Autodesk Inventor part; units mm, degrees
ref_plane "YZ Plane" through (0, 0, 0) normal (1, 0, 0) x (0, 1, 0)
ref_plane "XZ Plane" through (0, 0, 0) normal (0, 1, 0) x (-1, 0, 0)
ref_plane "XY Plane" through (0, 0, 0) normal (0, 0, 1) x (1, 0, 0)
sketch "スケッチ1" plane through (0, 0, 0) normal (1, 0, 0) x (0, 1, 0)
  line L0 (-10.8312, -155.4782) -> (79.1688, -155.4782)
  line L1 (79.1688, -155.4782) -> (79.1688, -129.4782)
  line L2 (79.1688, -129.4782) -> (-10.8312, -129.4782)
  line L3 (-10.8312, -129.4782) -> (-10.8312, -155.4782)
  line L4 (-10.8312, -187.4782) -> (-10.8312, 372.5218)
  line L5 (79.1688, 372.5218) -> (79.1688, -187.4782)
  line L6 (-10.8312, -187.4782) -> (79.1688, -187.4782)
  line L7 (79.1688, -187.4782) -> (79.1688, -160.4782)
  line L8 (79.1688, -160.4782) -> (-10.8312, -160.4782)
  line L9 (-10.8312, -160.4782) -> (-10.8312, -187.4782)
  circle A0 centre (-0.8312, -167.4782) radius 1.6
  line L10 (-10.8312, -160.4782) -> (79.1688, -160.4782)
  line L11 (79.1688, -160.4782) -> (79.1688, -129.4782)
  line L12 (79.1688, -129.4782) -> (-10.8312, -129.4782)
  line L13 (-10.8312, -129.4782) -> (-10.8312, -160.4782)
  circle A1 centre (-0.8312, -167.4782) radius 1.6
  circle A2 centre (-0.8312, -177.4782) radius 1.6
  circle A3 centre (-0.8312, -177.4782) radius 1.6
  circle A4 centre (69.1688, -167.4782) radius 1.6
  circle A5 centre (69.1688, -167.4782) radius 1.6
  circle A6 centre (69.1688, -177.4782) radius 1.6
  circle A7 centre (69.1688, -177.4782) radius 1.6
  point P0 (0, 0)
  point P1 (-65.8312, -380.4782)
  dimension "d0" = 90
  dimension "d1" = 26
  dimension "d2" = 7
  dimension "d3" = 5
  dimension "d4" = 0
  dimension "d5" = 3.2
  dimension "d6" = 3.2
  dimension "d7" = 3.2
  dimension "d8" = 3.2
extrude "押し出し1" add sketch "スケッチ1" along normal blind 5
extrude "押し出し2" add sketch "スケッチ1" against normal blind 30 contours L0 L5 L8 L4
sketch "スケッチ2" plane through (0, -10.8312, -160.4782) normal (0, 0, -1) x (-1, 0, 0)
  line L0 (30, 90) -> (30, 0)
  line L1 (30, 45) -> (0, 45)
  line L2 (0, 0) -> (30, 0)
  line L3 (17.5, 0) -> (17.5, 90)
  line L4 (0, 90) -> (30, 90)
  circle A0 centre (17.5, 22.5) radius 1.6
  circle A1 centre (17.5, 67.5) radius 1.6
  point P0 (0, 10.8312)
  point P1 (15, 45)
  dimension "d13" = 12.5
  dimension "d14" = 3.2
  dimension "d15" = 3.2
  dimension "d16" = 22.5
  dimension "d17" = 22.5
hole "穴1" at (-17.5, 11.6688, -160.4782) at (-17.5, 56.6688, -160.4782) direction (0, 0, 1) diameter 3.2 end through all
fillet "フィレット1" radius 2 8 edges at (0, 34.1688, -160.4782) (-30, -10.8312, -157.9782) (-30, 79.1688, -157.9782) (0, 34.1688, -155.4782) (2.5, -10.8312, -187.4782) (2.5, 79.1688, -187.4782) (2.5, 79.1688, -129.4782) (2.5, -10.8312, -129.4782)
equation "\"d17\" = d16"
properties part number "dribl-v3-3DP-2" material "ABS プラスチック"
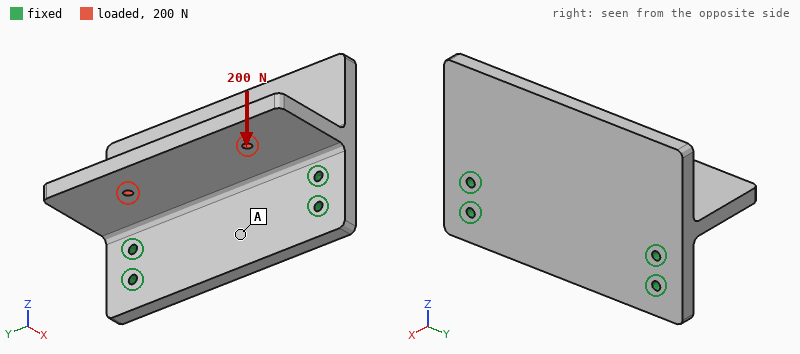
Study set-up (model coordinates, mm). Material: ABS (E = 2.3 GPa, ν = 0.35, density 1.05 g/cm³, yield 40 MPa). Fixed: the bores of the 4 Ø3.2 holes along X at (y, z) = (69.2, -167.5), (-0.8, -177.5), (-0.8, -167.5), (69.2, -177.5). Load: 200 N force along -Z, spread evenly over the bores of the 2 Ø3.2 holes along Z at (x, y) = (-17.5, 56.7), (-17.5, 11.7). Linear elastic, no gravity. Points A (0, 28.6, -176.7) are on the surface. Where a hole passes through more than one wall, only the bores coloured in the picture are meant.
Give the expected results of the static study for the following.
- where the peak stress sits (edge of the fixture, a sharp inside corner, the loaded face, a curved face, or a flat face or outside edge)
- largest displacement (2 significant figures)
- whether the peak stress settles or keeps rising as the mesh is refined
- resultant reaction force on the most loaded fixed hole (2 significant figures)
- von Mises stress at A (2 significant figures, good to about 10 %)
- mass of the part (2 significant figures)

edge of the fixture
1.1 mm
keeps rising
120 N
3.0 MPa
41 g
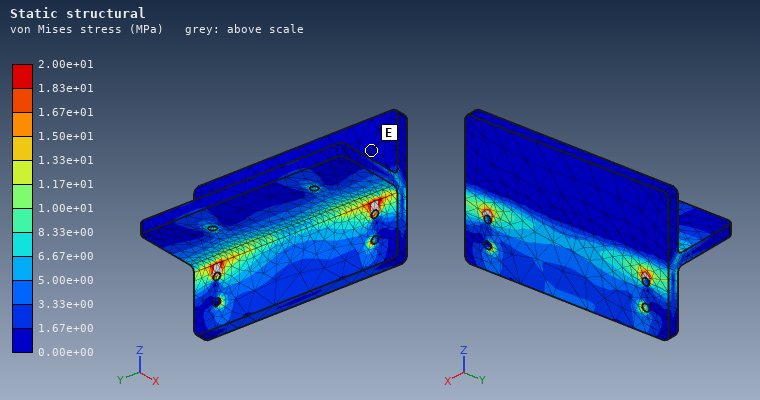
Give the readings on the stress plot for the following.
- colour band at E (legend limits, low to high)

0.00e+00 to 1.67e+00 MPa
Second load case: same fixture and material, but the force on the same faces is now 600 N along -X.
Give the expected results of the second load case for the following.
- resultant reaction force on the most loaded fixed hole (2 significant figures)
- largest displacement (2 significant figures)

400 N
0.86 mm
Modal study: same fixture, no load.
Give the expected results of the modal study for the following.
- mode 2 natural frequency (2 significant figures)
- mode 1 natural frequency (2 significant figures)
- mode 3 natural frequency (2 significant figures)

990 Hz
550 Hz
1400 Hz
